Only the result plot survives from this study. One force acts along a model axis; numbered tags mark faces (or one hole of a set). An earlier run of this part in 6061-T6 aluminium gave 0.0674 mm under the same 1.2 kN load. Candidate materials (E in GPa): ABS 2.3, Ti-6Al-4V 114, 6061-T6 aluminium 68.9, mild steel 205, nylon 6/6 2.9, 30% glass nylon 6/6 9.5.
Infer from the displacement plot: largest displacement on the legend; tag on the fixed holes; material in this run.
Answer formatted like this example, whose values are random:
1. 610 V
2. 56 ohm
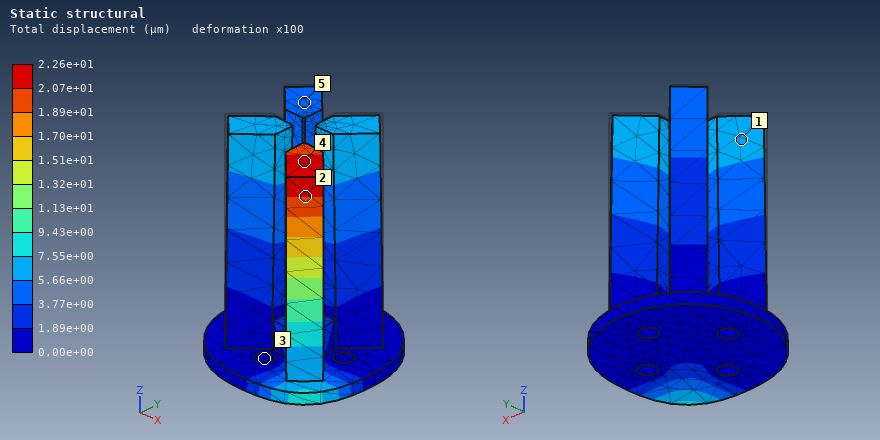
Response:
1. 2.26e+01 µm
2. 3
3. mild steel
